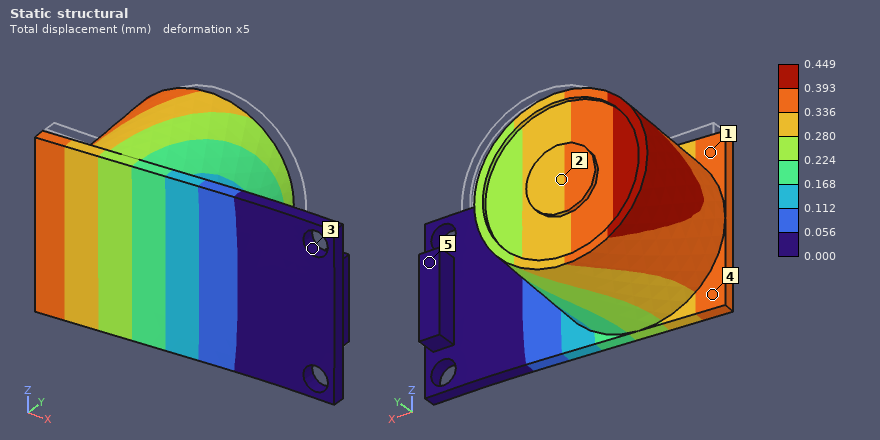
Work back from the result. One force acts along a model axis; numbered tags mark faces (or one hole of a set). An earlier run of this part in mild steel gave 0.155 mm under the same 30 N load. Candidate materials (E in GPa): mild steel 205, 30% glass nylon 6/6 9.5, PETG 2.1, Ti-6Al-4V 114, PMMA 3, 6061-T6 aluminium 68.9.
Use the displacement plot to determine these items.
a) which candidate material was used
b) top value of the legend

6061-T6 aluminium
0.449 mm
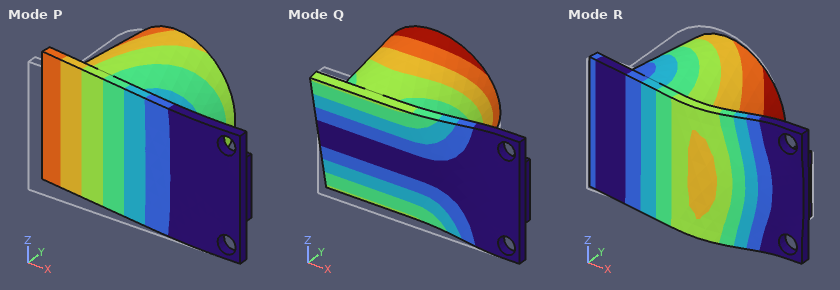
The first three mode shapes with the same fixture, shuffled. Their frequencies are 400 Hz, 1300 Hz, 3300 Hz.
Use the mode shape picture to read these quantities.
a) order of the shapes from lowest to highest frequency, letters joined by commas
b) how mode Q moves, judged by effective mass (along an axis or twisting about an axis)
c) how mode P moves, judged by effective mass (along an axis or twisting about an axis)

P, Q, R
along Z
along Y
